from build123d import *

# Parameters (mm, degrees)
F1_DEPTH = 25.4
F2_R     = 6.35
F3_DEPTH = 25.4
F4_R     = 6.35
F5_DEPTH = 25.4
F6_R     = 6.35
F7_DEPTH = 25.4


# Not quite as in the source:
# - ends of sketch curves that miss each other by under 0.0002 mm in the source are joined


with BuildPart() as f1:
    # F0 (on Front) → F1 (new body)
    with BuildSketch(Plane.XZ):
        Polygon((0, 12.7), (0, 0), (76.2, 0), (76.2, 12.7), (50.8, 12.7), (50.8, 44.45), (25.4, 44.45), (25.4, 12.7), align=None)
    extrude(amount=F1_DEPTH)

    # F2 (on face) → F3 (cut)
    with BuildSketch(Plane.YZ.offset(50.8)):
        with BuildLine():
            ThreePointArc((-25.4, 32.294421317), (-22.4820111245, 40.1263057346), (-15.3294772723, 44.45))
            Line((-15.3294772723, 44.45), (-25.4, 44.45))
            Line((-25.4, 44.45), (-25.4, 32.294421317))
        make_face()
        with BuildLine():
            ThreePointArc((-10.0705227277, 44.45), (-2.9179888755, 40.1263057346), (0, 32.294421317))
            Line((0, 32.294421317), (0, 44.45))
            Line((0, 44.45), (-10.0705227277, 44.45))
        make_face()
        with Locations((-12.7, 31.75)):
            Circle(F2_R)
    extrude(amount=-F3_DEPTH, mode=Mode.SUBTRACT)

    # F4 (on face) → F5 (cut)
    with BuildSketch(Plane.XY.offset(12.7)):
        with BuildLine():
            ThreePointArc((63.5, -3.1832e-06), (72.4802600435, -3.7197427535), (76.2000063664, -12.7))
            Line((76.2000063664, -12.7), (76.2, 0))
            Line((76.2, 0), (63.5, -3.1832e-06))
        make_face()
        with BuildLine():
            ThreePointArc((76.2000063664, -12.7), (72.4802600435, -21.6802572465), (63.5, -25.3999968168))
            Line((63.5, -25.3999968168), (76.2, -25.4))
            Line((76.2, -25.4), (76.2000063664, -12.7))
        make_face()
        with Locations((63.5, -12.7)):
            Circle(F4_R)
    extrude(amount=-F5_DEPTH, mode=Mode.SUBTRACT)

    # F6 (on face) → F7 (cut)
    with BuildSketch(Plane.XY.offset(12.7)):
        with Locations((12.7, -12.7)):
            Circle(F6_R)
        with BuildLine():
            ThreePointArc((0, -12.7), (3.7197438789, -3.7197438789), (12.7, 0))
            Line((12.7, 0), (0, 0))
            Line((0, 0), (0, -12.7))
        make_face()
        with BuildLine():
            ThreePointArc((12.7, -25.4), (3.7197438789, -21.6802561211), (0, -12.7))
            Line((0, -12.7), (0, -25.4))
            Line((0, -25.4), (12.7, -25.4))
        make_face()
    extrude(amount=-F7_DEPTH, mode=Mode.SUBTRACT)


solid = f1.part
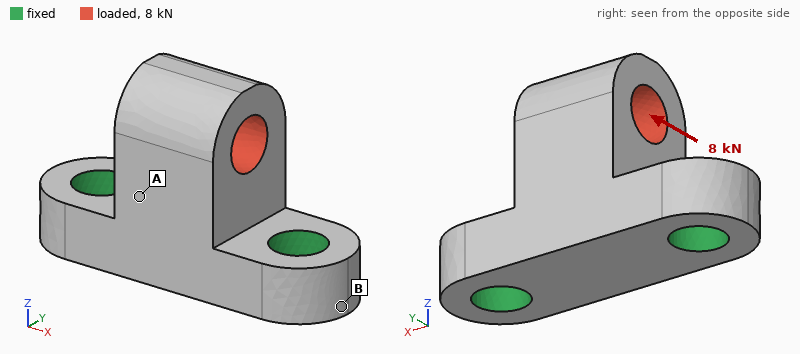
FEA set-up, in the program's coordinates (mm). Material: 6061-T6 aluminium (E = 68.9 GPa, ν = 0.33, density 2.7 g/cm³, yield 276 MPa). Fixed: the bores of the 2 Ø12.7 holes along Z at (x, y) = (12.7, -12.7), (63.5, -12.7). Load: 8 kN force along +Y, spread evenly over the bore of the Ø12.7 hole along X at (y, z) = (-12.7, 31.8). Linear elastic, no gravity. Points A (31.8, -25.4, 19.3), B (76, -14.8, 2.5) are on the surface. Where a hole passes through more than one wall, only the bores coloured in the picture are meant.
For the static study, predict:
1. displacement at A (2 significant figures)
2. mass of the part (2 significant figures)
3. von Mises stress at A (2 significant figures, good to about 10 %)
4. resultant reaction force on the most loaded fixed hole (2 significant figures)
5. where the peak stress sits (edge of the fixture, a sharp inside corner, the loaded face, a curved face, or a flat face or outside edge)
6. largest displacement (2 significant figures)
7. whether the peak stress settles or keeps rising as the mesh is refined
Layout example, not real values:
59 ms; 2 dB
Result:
0.075 mm; 95 g; 45 MPa; 4.0 kN; edge of the fixture; 0.18 mm; keeps rising
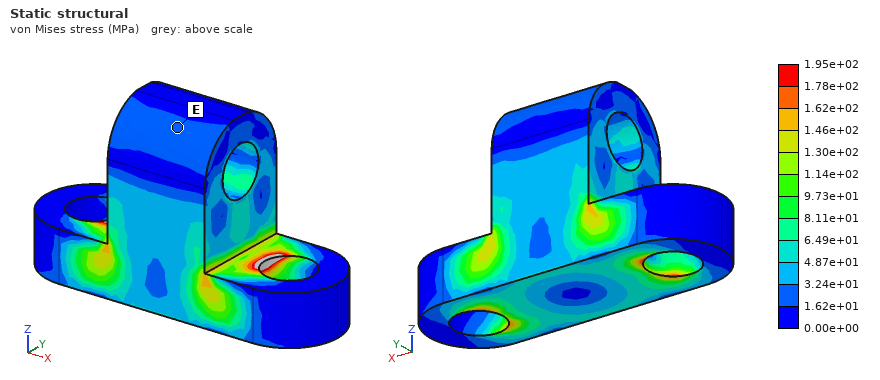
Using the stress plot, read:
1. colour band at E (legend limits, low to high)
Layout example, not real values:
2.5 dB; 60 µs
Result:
1.62e+01 to 3.24e+01 MPa
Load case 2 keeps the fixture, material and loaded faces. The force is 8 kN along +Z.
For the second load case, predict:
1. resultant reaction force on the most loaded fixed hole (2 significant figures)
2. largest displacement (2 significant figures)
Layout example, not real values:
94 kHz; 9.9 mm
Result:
4.2 kN; 18 µm
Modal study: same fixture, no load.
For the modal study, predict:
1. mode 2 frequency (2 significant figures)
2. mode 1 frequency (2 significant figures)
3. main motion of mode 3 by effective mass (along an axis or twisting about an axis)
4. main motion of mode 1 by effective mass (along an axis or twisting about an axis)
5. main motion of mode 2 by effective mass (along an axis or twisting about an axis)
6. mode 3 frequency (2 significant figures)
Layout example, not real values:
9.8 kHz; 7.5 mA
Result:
12 kHz; 6900 Hz; along Z; along Y; along X; 17 kHz
